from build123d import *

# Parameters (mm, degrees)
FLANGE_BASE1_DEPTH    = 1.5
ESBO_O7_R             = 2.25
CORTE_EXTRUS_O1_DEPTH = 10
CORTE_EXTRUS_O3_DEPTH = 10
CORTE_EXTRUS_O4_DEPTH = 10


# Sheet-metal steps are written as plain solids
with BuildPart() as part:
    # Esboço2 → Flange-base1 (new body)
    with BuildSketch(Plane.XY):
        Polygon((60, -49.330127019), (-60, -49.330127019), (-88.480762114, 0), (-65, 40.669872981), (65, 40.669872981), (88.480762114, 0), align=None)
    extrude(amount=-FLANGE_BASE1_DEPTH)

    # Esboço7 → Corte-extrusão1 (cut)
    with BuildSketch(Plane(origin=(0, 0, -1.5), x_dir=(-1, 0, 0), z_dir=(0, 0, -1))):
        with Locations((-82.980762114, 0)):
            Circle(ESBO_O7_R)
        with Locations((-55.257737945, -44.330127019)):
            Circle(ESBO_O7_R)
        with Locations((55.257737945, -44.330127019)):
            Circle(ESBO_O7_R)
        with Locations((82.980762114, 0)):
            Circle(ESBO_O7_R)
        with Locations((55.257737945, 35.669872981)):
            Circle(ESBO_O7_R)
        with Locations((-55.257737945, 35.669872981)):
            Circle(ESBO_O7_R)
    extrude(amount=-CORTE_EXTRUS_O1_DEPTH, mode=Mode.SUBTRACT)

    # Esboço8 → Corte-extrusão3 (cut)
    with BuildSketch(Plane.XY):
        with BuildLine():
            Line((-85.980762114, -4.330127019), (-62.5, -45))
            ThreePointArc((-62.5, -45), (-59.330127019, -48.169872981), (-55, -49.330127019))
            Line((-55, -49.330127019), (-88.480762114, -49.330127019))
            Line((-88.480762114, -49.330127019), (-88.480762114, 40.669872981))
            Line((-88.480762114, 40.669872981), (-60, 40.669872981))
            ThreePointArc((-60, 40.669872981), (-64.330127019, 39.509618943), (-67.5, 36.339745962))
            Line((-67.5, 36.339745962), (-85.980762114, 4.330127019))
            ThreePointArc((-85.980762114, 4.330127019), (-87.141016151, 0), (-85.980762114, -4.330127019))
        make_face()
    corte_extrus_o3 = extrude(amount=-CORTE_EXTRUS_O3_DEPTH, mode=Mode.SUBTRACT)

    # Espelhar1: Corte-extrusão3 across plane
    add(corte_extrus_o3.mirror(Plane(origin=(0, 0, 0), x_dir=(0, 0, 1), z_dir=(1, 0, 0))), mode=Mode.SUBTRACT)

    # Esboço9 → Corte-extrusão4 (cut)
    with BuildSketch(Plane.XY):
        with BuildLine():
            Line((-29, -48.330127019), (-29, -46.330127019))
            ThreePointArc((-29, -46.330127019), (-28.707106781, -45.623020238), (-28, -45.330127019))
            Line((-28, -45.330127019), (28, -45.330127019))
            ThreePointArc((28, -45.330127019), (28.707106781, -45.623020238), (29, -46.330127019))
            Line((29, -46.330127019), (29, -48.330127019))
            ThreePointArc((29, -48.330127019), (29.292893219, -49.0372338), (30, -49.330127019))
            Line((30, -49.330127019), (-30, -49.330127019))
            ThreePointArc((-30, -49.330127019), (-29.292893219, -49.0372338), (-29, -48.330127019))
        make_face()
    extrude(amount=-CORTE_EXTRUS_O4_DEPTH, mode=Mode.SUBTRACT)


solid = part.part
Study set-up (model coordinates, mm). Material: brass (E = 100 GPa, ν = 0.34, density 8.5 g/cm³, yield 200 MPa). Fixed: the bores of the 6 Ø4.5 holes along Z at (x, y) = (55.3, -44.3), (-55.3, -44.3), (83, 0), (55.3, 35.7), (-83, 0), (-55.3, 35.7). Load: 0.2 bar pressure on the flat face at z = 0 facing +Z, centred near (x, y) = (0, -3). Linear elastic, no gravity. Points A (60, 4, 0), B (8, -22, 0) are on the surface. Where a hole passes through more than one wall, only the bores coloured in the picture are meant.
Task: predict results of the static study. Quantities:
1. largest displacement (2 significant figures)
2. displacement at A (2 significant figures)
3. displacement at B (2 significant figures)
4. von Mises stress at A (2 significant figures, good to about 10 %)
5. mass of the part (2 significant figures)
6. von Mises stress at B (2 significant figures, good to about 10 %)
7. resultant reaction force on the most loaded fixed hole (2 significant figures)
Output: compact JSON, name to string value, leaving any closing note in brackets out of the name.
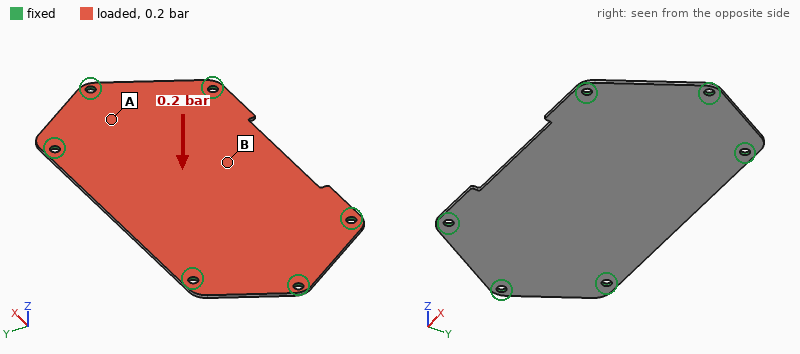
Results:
{"largest displacement": "0.41 mm", "displacement at A": "0.066 mm", "displacement at B": "0.39 mm", "von Mises stress at A": "16 MPa", "mass of the part": "170 g", "von Mises stress at B": "27 MPa", "resultant reaction force on the most loaded fixed hole": "61 N"}
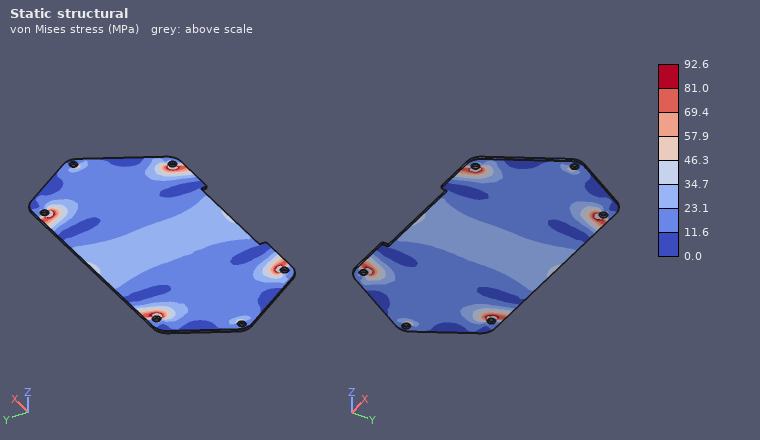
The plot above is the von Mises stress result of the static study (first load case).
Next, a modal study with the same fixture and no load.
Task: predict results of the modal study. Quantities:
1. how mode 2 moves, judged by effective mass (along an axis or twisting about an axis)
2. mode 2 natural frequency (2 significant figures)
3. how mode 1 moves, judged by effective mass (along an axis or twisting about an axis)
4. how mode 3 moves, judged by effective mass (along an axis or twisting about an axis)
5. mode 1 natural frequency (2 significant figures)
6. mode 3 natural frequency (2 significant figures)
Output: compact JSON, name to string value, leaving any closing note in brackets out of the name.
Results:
{"how mode 2 moves, judged by effective mass": "twisting about X", "mode 2 natural frequency": "590 Hz", "how mode 1 moves, judged by effective mass": "along Z", "how mode 3 moves, judged by effective mass": "twisting about Y", "mode 1 natural frequency": "370 Hz", "mode 3 natural frequency": "890 Hz"}
